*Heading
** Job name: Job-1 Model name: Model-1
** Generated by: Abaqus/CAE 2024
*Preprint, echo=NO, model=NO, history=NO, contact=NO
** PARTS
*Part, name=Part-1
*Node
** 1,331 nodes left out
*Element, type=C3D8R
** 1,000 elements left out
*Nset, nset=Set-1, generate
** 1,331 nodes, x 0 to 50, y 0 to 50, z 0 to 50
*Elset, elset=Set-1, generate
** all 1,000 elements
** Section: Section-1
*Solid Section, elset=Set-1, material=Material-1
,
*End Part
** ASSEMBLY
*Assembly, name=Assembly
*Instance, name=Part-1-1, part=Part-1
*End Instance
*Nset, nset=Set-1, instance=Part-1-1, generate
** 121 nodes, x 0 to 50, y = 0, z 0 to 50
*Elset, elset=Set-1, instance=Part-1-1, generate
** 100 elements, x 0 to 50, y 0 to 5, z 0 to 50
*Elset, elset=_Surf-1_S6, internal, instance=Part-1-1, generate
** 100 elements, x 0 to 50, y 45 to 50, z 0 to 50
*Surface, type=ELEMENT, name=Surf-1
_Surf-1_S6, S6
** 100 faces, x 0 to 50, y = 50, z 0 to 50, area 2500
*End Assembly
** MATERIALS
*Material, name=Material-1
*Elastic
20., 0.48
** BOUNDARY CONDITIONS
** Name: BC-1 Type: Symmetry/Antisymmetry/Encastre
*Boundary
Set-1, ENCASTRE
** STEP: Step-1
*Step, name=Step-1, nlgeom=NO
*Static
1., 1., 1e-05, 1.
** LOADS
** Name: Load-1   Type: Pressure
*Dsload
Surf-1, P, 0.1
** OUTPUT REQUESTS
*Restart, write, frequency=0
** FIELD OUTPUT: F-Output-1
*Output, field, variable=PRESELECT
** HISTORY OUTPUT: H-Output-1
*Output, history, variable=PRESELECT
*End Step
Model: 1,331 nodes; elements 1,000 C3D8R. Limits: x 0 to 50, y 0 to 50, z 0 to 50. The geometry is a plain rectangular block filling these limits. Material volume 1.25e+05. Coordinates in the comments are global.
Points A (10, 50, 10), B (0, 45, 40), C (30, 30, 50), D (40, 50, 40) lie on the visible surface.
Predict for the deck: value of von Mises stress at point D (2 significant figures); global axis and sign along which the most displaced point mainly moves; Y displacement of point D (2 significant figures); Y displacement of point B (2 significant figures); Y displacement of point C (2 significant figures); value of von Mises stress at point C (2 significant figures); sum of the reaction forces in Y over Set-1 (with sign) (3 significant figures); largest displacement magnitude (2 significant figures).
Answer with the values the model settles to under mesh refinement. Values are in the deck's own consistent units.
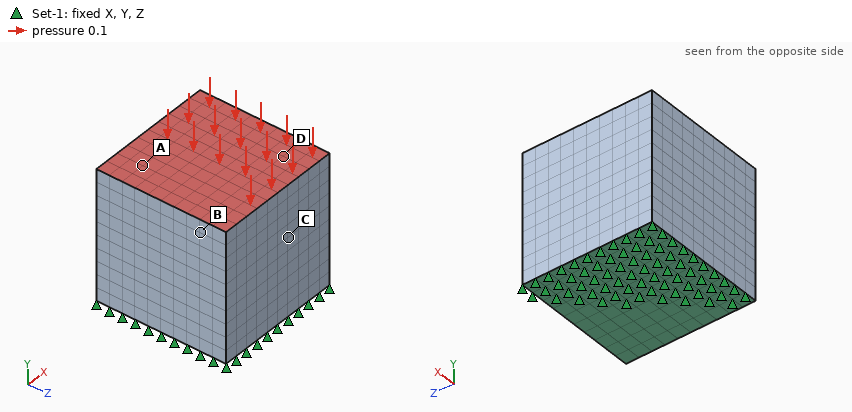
0.10
-Y
-0.23
-0.20
-0.13
0.098
250
0.25
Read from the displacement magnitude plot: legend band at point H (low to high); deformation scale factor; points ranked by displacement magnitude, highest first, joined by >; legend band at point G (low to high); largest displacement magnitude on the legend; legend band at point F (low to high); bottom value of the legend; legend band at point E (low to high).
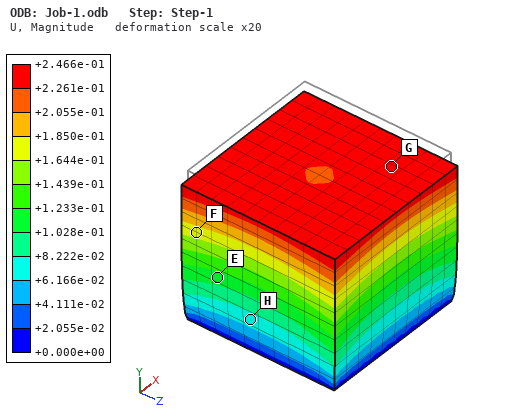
+6.166e-02 to +8.222e-02
20
G > F > E > H
+2.261e-01 to +2.466e-01
+2.466e-01
+1.644e-01 to +1.850e-01
+0.000e+00
+1.028e-01 to +1.233e-01
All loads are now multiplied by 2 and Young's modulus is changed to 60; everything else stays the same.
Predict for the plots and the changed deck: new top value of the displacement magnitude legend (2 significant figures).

0.16
